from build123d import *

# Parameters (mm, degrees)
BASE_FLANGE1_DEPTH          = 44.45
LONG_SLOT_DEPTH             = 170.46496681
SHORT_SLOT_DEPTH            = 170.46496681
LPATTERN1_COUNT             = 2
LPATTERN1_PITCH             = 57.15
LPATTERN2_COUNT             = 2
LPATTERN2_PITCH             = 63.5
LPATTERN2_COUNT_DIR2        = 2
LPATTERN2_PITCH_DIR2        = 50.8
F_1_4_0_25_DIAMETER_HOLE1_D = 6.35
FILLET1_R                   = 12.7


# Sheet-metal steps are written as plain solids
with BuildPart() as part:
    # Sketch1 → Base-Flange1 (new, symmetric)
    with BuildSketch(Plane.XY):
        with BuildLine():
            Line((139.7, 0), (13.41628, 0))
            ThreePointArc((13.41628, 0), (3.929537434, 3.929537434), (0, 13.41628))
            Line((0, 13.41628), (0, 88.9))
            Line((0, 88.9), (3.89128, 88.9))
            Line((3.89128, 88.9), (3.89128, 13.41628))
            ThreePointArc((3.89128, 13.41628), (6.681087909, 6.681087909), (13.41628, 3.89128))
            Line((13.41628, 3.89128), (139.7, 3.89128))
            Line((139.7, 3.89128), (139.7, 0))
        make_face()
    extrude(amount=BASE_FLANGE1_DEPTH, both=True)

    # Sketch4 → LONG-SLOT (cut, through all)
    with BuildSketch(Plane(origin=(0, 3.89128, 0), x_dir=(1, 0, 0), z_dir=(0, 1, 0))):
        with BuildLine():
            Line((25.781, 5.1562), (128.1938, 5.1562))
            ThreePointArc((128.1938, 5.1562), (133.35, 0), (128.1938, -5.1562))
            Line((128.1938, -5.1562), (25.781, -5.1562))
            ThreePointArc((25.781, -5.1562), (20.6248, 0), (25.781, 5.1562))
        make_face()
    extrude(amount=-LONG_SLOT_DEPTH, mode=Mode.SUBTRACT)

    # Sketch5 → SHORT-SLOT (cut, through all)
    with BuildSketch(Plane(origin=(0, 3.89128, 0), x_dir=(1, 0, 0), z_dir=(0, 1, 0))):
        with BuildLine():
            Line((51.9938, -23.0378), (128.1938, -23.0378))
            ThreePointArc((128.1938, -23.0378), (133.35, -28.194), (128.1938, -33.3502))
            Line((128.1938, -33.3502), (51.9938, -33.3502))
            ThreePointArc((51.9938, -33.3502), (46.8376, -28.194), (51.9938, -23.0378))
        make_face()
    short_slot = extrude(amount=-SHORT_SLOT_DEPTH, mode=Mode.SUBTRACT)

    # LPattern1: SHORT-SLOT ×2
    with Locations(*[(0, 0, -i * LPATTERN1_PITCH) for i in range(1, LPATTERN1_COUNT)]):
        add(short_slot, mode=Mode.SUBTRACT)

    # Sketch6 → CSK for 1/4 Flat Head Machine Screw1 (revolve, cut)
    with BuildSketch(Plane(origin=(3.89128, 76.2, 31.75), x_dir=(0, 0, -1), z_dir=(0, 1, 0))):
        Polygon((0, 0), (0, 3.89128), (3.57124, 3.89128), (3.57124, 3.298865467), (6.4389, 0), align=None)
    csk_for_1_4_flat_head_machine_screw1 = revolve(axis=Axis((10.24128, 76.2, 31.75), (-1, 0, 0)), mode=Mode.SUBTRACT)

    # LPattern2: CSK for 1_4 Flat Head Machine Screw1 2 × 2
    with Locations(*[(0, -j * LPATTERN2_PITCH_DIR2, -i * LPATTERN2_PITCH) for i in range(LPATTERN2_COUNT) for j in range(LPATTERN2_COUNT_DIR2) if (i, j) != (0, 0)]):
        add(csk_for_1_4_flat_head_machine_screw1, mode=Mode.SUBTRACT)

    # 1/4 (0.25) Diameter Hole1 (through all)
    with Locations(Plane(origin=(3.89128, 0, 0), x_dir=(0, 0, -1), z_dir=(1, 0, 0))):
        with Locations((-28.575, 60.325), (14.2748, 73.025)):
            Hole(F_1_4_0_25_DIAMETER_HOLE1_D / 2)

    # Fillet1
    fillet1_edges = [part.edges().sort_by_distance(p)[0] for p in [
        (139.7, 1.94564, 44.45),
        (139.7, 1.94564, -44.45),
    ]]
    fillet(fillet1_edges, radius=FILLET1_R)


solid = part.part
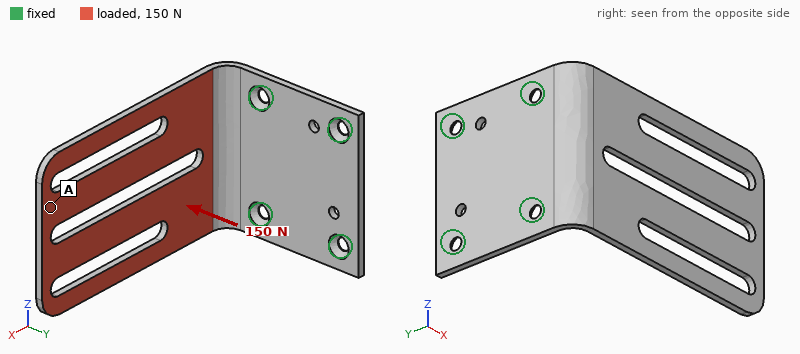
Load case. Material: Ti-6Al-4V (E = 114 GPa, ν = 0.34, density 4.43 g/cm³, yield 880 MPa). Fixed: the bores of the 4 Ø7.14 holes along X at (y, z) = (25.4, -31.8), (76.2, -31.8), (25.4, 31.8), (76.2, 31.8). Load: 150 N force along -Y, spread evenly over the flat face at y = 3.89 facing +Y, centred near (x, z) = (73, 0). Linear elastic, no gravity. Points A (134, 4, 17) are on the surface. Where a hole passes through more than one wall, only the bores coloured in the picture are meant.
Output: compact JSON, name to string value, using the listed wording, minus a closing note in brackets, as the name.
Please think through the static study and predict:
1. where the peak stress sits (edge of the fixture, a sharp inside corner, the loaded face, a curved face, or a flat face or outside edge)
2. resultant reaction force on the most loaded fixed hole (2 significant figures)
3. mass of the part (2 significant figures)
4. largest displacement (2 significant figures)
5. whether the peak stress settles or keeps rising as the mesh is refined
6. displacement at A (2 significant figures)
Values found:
{"where the peak stress sits": "edge of the fixture", "resultant reaction force on the most loaded fixed hole": "520 N", "mass of the part": "280 g", "largest displacement": "1.8 mm", "whether the peak stress settles or keeps rising as the mesh is refined": "keeps rising", "displacement at A": "1.7 mm"}
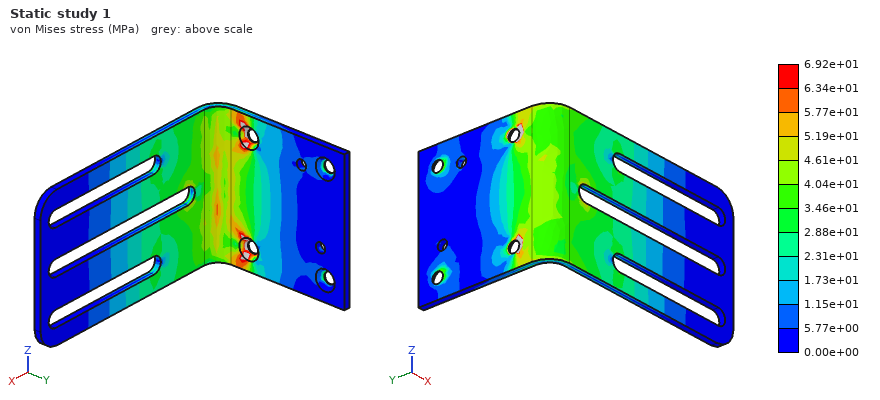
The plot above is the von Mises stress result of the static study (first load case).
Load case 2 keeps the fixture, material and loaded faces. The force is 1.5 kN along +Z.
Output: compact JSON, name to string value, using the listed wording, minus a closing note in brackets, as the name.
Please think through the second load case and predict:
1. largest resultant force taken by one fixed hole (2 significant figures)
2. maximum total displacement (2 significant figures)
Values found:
{"largest resultant force taken by one fixed hole": "3.1 kN", "maximum total displacement": "1.5 mm"}
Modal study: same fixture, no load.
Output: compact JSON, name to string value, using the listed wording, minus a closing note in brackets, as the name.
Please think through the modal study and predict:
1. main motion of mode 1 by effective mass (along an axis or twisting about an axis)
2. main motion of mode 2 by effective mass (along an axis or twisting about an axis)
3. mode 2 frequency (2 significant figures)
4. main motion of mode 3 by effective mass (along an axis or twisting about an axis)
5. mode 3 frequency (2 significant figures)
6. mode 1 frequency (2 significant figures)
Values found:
{"main motion of mode 1 by effective mass": "along Y", "main motion of mode 2 by effective mass": "along Z", "mode 2 frequency": "440 Hz", "main motion of mode 3 by effective mass": "along Z", "mode 3 frequency": "640 Hz", "mode 1 frequency": "150 Hz"}
